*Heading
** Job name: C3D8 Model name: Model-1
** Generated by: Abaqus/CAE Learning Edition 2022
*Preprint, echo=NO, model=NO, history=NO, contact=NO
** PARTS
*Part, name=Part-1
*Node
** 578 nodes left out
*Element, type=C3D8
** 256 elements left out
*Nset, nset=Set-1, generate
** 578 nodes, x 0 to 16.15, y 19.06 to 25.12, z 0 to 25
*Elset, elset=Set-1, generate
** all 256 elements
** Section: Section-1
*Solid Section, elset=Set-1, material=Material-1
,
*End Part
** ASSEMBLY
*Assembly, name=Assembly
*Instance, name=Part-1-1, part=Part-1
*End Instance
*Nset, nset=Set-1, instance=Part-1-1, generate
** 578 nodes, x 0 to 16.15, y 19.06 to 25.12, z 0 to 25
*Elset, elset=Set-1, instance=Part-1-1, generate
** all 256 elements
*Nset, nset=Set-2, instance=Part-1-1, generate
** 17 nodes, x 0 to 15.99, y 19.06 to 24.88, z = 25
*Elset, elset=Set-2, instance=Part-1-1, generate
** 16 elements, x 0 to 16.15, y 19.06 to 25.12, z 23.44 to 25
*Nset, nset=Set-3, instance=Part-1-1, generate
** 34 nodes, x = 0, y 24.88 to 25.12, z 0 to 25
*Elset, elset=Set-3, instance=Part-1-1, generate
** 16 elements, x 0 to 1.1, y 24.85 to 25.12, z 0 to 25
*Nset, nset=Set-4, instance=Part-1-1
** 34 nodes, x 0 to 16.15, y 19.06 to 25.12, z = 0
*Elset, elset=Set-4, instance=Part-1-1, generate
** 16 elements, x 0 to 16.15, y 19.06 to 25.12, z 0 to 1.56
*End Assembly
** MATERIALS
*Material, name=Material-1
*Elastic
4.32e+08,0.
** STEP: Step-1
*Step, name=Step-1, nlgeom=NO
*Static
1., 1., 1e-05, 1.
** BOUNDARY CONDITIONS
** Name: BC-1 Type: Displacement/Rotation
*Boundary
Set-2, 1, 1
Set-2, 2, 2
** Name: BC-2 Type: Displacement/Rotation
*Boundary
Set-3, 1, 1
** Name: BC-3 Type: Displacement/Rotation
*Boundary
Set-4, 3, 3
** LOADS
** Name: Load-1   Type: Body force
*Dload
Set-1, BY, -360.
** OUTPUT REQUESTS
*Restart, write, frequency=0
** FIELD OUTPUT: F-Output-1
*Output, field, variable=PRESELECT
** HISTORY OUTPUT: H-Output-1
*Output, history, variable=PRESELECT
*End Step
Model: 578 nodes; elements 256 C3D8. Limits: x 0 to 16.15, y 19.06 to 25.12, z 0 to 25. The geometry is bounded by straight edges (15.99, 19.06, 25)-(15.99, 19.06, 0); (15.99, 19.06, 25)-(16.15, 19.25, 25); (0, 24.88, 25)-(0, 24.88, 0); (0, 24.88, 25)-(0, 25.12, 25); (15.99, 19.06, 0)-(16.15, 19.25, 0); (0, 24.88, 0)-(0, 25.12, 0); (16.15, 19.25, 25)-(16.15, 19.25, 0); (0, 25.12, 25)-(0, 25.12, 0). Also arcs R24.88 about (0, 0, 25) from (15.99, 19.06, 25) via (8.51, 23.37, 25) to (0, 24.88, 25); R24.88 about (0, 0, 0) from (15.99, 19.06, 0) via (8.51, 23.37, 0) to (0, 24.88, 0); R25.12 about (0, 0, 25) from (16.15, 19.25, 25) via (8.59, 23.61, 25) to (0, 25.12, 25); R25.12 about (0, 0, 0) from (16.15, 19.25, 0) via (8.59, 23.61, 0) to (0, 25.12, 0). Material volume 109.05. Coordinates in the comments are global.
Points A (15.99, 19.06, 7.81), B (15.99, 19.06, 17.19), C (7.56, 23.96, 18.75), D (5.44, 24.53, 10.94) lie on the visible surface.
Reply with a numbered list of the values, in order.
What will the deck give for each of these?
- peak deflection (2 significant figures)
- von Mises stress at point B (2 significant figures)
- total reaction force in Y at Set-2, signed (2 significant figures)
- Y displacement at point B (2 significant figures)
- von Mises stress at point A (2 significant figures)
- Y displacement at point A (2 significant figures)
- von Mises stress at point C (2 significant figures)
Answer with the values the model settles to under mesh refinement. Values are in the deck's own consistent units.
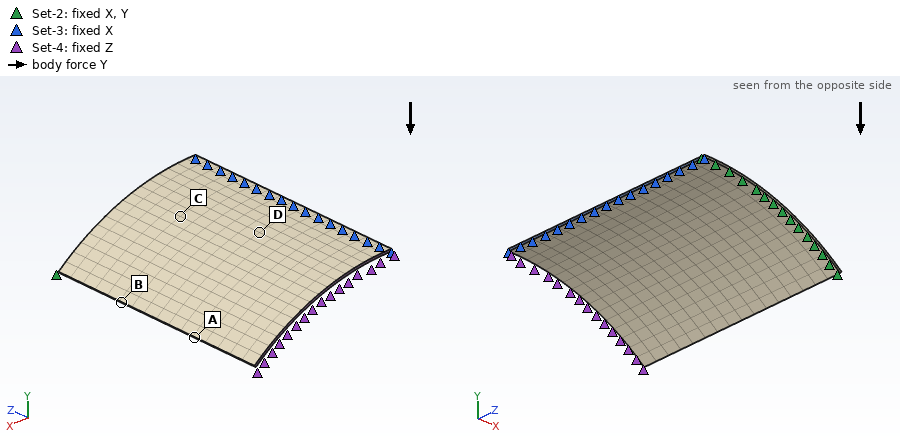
1. 0.34
2. 2.7e+05
3. 39000
4. -0.15
5. 3.4e+05
6. -0.27
7. 1.7e+05
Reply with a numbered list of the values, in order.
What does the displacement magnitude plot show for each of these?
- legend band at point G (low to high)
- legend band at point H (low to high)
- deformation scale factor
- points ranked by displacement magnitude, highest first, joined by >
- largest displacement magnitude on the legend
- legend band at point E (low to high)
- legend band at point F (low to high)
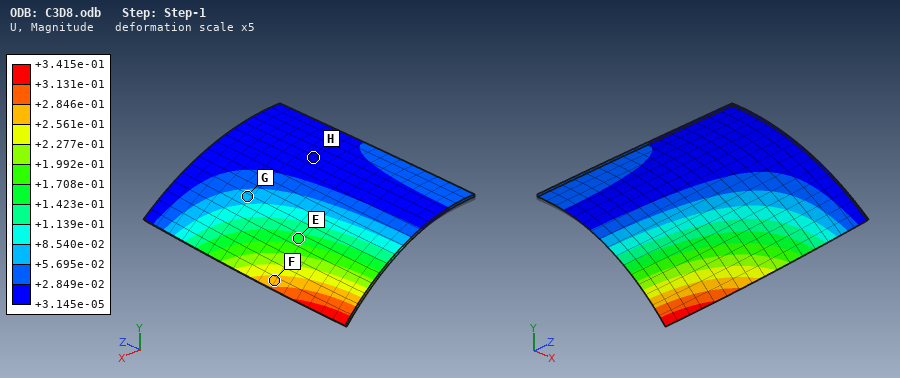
1. +5.695e-02 to +8.540e-02
2. +3.145e-05 to +2.849e-02
3. 5
4. F > E > G > H
5. +3.415e-01
6. +1.423e-01 to +1.708e-01
7. +2.561e-01 to +2.846e-01
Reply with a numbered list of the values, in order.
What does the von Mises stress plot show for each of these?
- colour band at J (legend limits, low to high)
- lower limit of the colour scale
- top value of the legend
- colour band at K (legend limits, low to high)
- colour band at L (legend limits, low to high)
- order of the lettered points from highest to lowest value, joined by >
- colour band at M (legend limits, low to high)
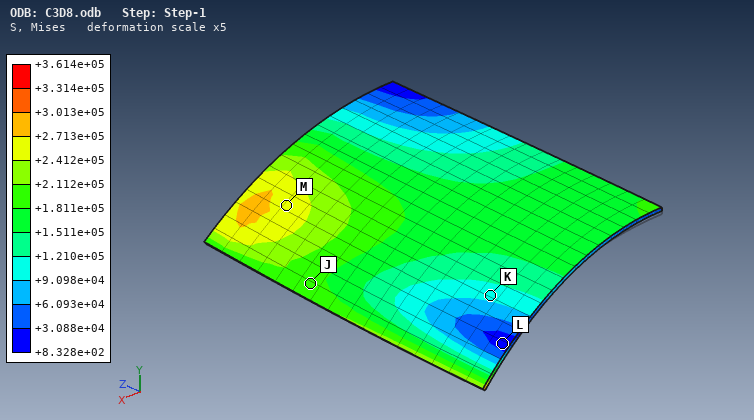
1. +1.811e+05 to +2.112e+05
2. +8.328e+02
3. +3.614e+05
4. +9.098e+04 to +1.210e+05
5. +8.328e+02 to +3.088e+04
6. M > J > K > L
7. +2.412e+05 to +2.713e+05
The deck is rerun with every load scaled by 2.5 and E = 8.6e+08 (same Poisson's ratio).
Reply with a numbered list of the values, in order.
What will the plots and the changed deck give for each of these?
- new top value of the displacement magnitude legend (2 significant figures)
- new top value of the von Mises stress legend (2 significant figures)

1. 0.43
2. 9.0e+05
